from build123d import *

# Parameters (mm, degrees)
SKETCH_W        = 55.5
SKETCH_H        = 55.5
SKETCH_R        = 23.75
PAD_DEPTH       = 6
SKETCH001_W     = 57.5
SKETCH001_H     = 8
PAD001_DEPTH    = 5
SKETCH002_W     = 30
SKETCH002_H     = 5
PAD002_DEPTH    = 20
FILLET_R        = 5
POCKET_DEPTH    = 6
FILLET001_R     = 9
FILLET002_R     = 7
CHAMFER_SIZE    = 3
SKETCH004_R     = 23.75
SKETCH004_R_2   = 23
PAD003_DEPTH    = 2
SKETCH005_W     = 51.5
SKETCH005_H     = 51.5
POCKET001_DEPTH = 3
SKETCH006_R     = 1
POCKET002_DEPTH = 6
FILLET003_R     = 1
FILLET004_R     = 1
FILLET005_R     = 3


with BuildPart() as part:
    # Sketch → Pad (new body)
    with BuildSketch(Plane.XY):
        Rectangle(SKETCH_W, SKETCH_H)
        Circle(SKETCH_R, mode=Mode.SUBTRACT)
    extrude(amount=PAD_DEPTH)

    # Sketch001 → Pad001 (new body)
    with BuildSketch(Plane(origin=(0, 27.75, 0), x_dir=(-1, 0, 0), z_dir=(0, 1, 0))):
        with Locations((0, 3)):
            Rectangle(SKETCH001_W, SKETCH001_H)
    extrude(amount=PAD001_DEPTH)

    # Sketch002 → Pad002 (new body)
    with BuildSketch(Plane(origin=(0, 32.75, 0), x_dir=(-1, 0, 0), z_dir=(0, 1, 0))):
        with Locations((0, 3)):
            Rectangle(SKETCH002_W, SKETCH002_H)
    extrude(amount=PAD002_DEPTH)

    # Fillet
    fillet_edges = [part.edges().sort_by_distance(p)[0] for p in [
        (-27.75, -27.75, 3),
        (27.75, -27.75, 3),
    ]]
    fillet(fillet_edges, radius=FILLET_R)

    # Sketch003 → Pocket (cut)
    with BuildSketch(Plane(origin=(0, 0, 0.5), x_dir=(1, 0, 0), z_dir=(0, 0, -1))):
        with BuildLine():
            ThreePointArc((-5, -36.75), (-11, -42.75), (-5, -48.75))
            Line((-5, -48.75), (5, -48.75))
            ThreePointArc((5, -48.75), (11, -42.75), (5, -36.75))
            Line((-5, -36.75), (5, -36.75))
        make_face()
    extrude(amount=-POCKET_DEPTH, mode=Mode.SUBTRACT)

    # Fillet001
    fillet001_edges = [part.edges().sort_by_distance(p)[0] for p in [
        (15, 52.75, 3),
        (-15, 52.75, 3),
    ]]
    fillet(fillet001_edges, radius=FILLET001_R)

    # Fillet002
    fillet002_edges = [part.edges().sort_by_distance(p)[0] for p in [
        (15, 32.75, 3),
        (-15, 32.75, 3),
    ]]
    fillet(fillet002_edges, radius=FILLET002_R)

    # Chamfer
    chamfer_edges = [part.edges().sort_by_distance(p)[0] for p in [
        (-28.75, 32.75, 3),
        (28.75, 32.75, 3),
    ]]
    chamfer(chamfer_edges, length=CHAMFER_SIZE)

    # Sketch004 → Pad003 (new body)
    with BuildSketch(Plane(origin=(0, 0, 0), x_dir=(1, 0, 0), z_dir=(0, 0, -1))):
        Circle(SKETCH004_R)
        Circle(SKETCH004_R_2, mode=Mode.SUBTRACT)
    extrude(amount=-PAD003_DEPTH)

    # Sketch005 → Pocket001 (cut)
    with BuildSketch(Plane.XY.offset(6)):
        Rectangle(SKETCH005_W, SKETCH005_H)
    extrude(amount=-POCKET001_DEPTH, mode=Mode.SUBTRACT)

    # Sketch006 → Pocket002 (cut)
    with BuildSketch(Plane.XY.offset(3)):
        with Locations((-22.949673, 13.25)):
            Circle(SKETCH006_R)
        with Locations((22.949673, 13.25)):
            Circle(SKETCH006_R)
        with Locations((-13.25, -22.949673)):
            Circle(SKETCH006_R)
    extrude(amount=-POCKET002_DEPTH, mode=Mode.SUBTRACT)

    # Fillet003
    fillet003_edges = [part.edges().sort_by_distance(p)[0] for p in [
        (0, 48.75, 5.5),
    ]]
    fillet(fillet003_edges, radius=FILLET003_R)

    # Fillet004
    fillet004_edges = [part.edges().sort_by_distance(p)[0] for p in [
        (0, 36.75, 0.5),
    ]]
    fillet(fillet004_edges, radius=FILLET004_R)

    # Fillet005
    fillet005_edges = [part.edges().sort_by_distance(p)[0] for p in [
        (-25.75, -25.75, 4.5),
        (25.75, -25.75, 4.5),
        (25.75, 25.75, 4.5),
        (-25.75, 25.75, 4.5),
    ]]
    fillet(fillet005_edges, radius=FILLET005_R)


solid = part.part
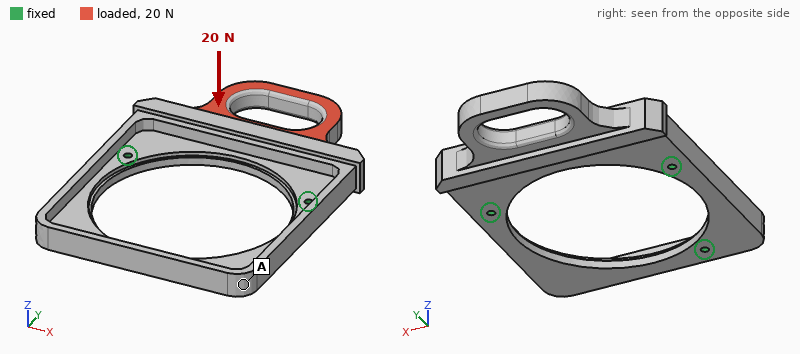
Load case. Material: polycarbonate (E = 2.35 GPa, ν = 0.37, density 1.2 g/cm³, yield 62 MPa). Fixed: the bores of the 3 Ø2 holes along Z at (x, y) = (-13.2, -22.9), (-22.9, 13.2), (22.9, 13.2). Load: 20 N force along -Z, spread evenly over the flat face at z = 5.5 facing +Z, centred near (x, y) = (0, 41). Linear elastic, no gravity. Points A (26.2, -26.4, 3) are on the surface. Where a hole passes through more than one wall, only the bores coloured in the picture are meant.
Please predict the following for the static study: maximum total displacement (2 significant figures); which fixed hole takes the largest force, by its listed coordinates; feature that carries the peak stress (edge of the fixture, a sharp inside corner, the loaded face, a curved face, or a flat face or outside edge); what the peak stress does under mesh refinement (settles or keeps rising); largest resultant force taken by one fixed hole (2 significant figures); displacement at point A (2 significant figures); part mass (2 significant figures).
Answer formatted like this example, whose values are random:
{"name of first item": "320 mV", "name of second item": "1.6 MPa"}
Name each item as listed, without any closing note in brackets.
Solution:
{"maximum total displacement": "1.00 mm", "which fixed hole takes the largest force, by its listed coordinates": "(-22.9, 13.2)", "feature that carries the peak stress": "edge of the fixture", "what the peak stress does under mesh refinement": "keeps rising", "largest resultant force taken by one fixed hole": "14 N", "displacement at point A": "0.15 mm", "part mass": "11 g"}
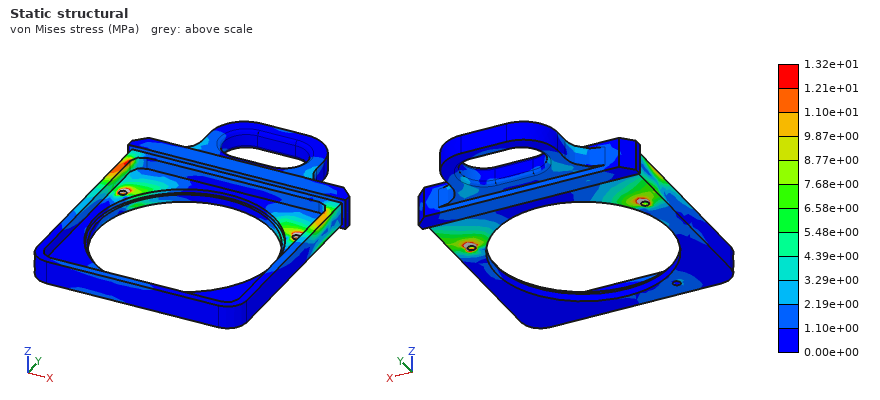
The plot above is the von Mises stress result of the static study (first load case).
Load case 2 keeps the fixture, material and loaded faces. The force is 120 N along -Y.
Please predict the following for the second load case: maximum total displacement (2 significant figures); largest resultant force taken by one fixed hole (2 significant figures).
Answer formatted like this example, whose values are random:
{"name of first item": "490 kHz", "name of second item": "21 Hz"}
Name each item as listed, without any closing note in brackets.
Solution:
{"maximum total displacement": "1.1 mm", "largest resultant force taken by one fixed hole": "67 N"}
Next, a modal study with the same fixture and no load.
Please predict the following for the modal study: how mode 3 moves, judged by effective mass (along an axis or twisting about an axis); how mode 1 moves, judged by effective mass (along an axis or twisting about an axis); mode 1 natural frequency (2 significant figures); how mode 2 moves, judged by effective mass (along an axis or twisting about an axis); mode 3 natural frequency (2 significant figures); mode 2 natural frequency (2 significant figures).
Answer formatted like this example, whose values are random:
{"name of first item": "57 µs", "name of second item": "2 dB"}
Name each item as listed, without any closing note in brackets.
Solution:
{"how mode 3 moves, judged by effective mass": "twisting about Y", "how mode 1 moves, judged by effective mass": "along Z", "mode 1 natural frequency": "490 Hz", "how mode 2 moves, judged by effective mass": "along Z", "mode 3 natural frequency": "1800 Hz", "mode 2 natural frequency": "720 Hz"}
